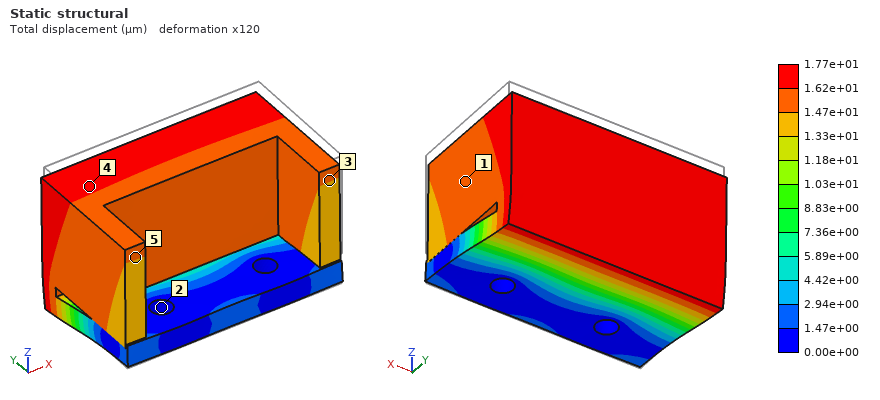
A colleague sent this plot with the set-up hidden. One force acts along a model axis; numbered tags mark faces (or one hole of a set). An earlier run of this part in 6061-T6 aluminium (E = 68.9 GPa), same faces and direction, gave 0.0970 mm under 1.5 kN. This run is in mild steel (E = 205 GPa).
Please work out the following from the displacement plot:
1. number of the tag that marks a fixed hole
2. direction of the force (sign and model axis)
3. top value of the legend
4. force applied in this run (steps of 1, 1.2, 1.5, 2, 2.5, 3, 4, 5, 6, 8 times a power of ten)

2
-Z
1.77e+01 µm
800 N
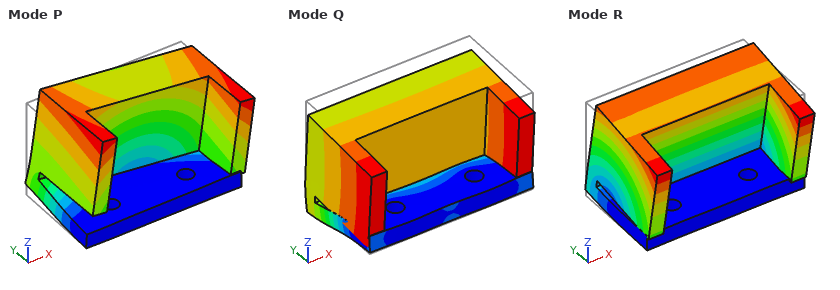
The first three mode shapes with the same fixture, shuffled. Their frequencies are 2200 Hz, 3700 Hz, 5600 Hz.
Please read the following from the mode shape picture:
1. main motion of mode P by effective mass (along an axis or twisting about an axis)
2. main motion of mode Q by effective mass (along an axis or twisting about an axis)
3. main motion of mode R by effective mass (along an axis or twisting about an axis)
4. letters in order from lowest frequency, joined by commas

along X
along Z
along Y
R, P, Q
